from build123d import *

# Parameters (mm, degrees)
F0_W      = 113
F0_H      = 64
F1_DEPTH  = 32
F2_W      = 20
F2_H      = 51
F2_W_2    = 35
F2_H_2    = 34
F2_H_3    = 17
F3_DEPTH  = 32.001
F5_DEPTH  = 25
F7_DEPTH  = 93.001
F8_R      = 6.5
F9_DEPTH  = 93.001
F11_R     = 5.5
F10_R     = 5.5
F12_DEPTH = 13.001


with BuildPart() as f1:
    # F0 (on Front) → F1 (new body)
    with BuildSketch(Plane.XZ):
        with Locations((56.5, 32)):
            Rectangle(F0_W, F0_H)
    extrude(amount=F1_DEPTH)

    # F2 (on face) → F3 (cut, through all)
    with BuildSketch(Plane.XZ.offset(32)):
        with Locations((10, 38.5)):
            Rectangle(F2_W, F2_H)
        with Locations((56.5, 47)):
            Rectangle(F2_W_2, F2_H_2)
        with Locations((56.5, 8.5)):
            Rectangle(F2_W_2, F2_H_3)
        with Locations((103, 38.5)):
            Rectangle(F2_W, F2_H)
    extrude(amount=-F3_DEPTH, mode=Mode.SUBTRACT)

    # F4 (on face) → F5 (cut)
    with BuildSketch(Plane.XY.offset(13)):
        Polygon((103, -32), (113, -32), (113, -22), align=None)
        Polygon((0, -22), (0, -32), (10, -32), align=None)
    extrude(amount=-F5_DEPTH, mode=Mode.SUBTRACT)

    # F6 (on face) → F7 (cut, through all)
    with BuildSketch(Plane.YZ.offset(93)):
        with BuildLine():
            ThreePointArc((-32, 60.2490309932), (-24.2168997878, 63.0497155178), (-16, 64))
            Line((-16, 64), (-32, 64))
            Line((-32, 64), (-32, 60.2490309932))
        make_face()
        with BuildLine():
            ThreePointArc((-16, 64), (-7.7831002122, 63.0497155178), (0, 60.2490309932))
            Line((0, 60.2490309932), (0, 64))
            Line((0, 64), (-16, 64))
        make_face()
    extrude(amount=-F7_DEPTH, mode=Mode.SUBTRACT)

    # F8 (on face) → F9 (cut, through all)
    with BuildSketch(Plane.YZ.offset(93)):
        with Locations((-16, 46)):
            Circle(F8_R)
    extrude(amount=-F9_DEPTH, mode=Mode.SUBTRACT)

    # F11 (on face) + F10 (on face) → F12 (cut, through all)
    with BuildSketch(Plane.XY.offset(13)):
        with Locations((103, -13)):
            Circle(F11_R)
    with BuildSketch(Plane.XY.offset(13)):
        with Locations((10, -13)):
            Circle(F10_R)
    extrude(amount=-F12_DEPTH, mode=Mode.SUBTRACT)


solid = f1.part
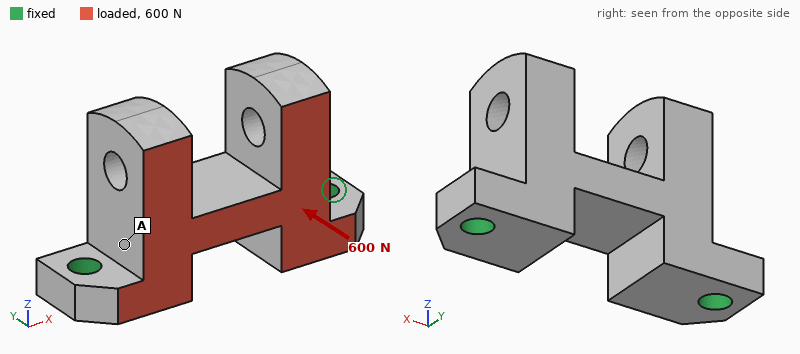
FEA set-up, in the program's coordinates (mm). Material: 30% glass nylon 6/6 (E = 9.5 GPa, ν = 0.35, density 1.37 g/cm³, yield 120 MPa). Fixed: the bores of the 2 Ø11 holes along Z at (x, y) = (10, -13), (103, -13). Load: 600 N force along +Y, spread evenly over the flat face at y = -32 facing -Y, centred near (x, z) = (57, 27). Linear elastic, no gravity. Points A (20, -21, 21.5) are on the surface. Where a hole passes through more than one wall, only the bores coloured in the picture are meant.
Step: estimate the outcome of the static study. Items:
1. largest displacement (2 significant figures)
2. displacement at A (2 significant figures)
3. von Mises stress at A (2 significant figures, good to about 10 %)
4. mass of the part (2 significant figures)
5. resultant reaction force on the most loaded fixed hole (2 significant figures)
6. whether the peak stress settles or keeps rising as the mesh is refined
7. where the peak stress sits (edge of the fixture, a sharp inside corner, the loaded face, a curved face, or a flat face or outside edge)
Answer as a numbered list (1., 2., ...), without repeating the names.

1. 75 µm
2. 22 µm
3. 1.6 MPa
4. 140 g
5. 300 N
6. keeps rising
7. edge of the fixture
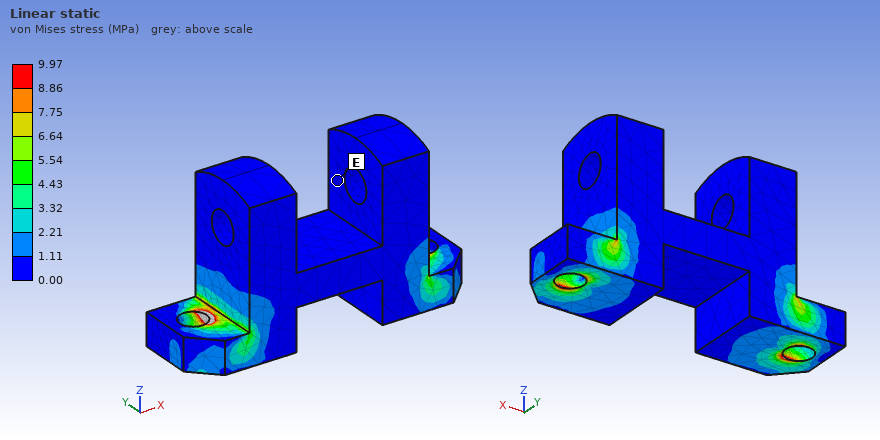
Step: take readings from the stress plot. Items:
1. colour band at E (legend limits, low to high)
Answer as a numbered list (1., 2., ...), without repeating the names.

1. 0.00 to 1.11 MPa
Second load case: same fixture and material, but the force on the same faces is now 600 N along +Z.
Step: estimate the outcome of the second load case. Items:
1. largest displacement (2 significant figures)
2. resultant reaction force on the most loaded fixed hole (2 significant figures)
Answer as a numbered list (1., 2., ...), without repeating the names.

1. 59 µm
2. 350 N
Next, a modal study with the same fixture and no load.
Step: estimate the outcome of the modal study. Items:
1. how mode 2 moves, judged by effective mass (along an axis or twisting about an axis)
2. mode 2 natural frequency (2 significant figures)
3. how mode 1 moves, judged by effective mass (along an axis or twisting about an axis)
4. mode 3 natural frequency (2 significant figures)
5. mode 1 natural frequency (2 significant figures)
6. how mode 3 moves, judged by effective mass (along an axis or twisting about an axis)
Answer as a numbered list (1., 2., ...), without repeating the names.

1. twisting about Z
2. 2300 Hz
3. along Y
4. 2900 Hz
5. 1500 Hz
6. along X
